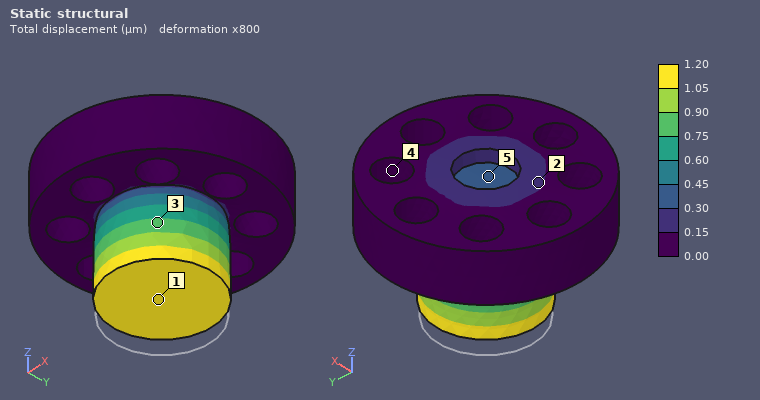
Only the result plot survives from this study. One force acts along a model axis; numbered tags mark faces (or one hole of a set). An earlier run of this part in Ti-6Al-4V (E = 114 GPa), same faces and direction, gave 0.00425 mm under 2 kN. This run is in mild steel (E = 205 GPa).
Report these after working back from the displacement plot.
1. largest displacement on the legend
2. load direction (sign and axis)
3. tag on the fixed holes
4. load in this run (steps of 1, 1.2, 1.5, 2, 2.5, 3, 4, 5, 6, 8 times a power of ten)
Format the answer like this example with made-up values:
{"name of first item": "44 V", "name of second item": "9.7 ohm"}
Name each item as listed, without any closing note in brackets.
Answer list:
{"largest displacement on the legend": "1.20 µm", "load direction": "+Z", "tag on the fixed holes": "4", "load in this run": "1 kN"}
